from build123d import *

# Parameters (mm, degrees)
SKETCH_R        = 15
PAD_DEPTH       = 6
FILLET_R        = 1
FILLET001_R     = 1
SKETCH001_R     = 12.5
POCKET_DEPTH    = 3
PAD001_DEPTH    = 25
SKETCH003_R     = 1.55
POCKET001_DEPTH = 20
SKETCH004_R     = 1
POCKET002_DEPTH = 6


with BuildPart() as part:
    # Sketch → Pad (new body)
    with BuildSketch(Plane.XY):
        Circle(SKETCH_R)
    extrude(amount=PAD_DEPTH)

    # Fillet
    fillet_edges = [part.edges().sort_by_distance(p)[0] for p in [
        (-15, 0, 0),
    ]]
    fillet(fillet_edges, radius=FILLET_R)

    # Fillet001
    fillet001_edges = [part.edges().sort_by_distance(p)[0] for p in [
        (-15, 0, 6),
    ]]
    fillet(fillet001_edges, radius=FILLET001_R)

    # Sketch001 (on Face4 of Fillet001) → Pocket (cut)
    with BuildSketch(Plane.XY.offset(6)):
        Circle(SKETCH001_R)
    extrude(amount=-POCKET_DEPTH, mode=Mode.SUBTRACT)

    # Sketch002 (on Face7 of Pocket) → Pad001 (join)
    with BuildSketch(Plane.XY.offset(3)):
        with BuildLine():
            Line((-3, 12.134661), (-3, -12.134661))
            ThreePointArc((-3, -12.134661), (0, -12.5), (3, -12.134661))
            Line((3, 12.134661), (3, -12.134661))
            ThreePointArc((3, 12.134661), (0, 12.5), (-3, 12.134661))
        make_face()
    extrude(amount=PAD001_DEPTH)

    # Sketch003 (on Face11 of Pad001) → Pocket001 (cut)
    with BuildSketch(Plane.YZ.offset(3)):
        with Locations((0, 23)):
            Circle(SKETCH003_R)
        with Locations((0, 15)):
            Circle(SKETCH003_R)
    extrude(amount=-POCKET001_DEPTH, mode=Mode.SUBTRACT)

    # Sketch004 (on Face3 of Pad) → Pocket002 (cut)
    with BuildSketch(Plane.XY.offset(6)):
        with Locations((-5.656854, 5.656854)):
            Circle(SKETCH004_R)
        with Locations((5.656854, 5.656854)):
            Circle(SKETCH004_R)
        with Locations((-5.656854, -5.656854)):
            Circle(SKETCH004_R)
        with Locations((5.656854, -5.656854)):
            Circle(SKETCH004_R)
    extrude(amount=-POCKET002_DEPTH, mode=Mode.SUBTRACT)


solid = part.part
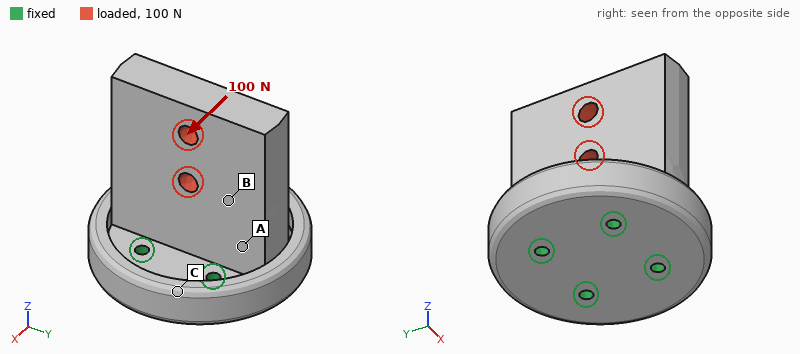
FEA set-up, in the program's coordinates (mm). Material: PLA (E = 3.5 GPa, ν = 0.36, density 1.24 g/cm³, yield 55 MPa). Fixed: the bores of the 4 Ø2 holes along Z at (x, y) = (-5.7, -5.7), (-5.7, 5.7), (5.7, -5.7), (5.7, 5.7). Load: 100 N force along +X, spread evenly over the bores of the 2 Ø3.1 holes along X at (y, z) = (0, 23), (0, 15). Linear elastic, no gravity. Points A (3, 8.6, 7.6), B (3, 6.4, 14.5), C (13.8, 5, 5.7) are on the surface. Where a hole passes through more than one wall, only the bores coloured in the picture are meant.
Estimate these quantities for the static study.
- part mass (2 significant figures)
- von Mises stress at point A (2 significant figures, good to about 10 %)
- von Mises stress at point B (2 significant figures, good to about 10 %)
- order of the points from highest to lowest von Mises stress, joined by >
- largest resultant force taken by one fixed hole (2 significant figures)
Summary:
7.8 g
7.3 MPa
3.5 MPa
A > B > C
87 N
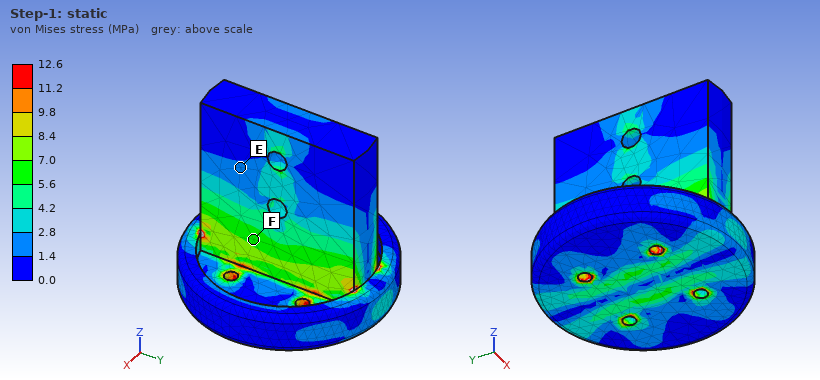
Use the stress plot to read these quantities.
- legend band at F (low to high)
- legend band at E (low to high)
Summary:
5.6 to 7.0 MPa
1.4 to 2.8 MPa
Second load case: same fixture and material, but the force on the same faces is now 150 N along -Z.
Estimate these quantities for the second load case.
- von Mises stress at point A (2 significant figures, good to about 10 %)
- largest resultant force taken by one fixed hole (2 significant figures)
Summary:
0.92 MPa
39 N
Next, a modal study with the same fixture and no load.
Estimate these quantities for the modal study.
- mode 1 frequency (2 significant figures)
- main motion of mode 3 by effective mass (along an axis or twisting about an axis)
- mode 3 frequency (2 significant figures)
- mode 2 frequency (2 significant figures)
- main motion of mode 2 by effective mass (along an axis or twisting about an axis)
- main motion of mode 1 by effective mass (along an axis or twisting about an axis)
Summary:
2100 Hz
twisting about Z
4900 Hz
3500 Hz
along Y
along X
